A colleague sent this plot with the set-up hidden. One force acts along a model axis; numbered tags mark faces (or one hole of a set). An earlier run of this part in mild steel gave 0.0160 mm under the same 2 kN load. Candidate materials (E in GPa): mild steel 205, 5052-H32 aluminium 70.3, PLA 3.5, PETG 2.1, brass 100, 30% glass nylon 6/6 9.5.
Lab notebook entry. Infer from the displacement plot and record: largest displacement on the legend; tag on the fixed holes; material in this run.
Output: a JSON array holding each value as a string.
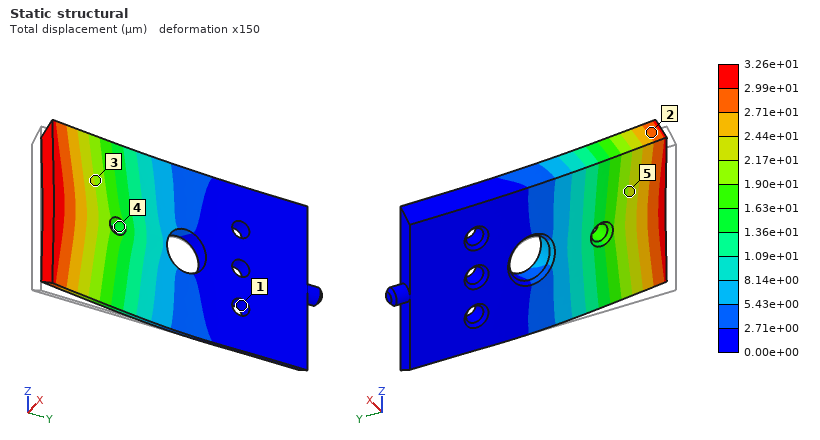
["3.26e+01 µm", "1", "brass"]
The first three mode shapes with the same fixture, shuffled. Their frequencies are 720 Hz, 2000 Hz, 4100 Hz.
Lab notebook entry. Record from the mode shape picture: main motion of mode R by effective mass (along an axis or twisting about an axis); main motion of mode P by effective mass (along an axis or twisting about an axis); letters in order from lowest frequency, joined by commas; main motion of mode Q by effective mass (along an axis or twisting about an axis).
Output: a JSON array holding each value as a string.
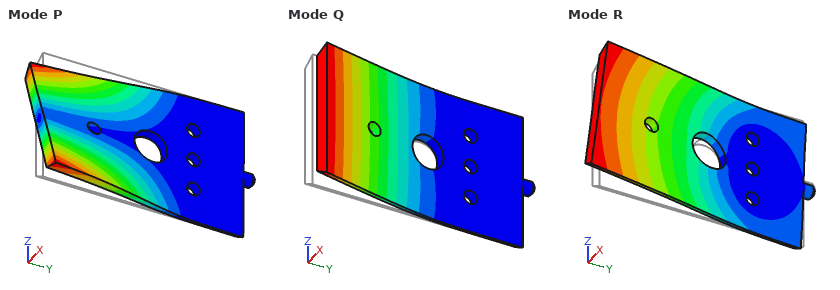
["along Z", "twisting about Y", "Q, P, R", "along X"]
